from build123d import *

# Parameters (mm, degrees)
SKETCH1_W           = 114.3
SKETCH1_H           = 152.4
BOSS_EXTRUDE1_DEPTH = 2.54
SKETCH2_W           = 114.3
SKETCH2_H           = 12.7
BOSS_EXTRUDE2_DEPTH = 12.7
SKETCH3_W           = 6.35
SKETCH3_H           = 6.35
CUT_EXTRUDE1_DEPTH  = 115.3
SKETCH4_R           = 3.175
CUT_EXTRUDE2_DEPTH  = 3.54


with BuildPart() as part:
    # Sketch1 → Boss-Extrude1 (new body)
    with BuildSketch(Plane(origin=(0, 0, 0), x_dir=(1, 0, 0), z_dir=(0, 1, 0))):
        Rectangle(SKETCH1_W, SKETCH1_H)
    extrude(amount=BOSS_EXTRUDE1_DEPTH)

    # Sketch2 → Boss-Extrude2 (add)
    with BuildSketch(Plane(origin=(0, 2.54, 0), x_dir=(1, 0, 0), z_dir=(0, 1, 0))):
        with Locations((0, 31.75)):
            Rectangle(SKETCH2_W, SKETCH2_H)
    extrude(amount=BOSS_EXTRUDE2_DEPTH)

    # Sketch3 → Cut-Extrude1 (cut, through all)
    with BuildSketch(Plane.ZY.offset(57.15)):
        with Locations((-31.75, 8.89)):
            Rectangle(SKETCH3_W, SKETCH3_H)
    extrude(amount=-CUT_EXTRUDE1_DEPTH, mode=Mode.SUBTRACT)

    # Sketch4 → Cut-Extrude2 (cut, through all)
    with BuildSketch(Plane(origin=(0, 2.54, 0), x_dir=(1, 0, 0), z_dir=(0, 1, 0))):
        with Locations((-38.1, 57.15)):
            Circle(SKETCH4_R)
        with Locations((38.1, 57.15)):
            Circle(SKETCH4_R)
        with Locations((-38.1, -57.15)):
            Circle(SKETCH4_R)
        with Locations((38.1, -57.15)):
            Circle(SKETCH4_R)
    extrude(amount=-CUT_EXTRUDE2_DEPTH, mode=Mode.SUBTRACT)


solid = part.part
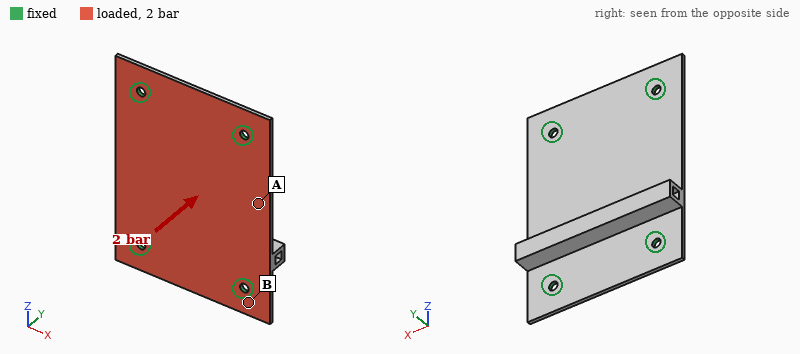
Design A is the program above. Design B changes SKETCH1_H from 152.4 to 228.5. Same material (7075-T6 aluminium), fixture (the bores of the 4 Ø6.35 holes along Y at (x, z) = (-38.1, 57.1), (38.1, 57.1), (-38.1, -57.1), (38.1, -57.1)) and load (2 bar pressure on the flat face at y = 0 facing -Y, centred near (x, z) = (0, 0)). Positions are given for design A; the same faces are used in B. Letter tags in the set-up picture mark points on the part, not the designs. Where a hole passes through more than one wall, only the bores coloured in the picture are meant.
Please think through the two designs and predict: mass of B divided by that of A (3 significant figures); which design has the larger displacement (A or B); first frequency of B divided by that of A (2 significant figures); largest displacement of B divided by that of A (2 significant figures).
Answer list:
1.38
B
0.70
2.9
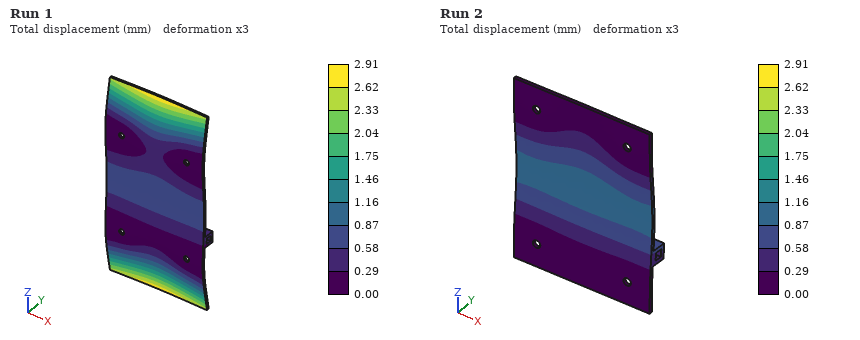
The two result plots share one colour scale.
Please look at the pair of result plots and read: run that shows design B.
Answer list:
Run 1
